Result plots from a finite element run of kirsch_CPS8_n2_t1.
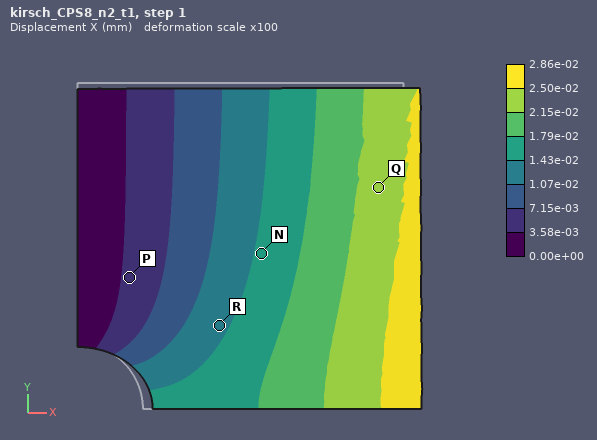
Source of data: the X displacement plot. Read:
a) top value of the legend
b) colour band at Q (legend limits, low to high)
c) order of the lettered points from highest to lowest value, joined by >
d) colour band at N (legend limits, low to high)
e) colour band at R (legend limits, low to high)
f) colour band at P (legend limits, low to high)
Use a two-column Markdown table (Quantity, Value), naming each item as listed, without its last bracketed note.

| Quantity | Value |
|---|---|
| top value of the legend | 2.86e-02 mm |
| colour band at Q | 2.15e-02 to 2.50e-02 mm |
| order of the lettered points from highest to lowest value, joined by > | Q > N > R > P |
| colour band at N | 1.43e-02 to 1.79e-02 mm |
| colour band at R | 1.07e-02 to 1.43e-02 mm |
| colour band at P | 3.58e-03 to 7.15e-03 mm |
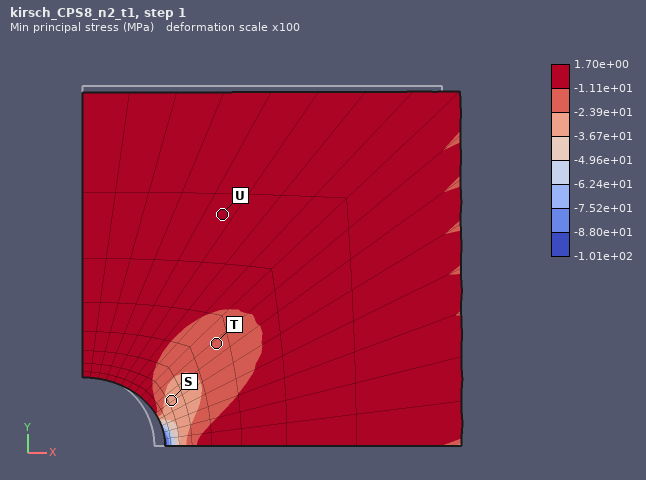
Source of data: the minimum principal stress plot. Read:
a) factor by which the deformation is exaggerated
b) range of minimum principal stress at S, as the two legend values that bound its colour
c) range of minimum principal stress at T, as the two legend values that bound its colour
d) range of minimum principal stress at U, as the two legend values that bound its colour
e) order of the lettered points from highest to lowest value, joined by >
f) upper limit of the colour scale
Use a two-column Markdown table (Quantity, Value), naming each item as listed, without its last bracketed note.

| Quantity | Value |
|---|---|
| factor by which the deformation is exaggerated | 100 |
| range of minimum principal stress at S, as the two legend values that bound its colour | -3.67e+01 to -2.39e+01 MPa |
| range of minimum principal stress at T, as the two legend values that bound its colour | -2.39e+01 to -1.11e+01 MPa |
| range of minimum principal stress at U, as the two legend values that bound its colour | -1.11e+01 to 1.70e+00 MPa |
| order of the lettered points from highest to lowest value, joined by > | U > T > S |
| upper limit of the colour scale | 1.70e+00 MPa |
